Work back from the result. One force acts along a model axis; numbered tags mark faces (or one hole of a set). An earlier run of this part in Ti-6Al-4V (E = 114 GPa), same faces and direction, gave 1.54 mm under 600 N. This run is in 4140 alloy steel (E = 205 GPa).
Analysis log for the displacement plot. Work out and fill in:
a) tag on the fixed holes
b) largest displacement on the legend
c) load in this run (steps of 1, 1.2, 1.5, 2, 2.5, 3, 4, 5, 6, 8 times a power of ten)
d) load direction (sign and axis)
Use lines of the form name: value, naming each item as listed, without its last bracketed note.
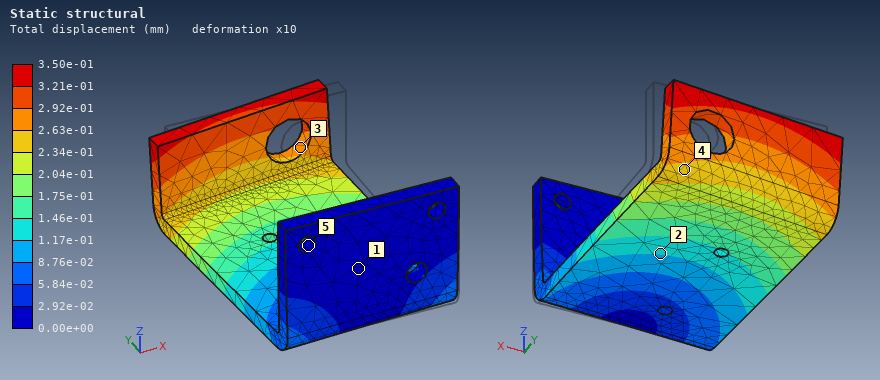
tag on the fixed holes: 5
largest displacement on the legend: 3.50e-01 mm
load in this run: 250 N
load direction: -X
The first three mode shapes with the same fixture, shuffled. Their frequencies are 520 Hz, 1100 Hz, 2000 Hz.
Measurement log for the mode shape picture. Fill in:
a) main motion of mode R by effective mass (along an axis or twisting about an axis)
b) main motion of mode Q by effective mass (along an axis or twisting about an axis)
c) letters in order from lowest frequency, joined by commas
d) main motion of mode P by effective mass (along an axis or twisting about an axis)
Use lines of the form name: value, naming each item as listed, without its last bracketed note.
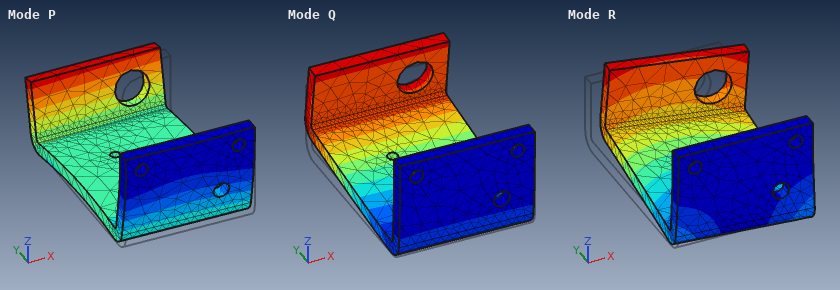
main motion of mode R by effective mass: along X
main motion of mode Q by effective mass: along Z
letters in order from lowest frequency, joined by commas: Q, R, P
main motion of mode P by effective mass: along Y
